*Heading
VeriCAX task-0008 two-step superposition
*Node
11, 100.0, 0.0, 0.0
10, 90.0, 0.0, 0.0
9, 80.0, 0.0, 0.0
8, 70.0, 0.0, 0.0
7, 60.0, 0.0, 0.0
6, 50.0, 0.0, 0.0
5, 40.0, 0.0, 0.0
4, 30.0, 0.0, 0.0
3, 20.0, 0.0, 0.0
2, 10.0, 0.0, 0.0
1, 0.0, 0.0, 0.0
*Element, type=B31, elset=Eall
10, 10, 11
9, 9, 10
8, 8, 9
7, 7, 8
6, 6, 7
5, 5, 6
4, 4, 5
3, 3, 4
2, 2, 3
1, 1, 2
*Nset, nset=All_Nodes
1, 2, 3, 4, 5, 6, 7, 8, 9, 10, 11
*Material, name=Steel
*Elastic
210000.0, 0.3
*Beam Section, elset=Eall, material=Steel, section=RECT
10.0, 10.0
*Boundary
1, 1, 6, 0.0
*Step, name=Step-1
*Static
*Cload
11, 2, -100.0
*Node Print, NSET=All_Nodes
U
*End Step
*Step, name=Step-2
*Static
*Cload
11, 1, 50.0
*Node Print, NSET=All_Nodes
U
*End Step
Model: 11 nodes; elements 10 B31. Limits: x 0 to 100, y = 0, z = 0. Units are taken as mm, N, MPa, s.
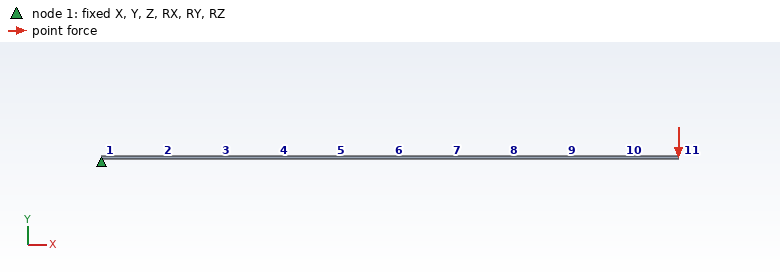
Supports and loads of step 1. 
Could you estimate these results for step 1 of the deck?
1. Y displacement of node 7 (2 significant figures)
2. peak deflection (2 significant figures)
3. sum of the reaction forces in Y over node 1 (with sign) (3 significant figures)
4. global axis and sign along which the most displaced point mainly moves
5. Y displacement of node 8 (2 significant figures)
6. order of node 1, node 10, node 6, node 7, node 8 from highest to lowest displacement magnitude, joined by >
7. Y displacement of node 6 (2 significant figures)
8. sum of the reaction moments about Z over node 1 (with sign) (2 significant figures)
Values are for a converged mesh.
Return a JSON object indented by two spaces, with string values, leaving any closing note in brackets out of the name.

{
  "Y displacement of node 7": "-0.083 mm",
  "peak deflection": "0.19 mm",
  "sum of the reaction forces in Y over node 1 (with sign)": "100 N",
  "global axis and sign along which the most displaced point mainly moves": "-Y",
  "Y displacement of node 8": "-0.11 mm",
  "order of node 1, node 10, node 6, node 7, node 8 from highest to lowest displacement magnitude, joined by >": "node 10 > node 8 > node 7 > node 6 > node 1",
  "Y displacement of node 6": "-0.060 mm",
  "sum of the reaction moments about Z over node 1 (with sign)": "10000 N·mm"
}
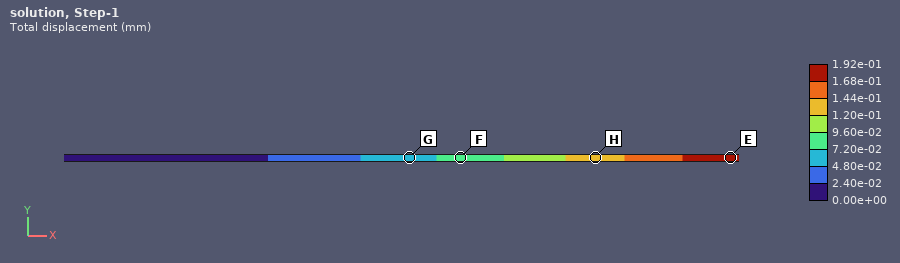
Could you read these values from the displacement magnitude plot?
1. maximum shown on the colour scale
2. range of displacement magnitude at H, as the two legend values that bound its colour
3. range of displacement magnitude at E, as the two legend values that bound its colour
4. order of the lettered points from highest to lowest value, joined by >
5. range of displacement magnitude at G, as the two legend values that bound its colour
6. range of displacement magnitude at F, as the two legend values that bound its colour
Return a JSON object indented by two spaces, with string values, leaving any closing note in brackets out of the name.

{
  "maximum shown on the colour scale": "1.92e-01 mm",
  "range of displacement magnitude at H, as the two legend values that bound its colour": "1.20e-01 to 1.44e-01 mm",
  "range of displacement magnitude at E, as the two legend values that bound its colour": "1.68e-01 to 1.92e-01 mm",
  "order of the lettered points from highest to lowest value, joined by >": "E > H > F > G",
  "range of displacement magnitude at G, as the two legend values that bound its colour": "4.80e-02 to 7.20e-02 mm",
  "range of displacement magnitude at F, as the two legend values that bound its colour": "7.20e-02 to 9.60e-02 mm"
}
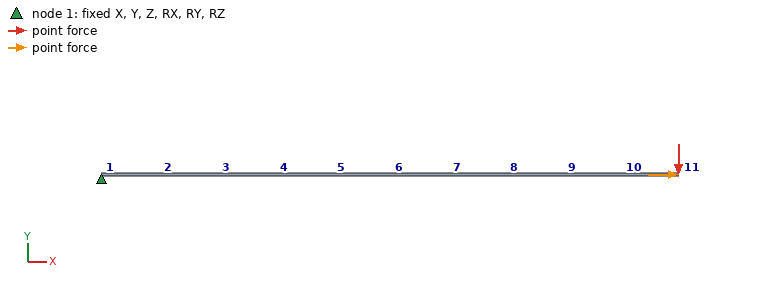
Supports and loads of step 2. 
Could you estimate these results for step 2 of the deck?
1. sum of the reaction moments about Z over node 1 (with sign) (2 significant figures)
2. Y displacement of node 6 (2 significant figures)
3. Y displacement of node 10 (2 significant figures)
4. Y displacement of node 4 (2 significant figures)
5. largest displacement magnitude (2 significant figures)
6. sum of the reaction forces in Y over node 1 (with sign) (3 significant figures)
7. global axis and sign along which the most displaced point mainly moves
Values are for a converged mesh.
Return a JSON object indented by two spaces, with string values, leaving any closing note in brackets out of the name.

{
  "sum of the reaction moments about Z over node 1 (with sign)": "10000 N·mm",
  "Y displacement of node 6": "-0.060 mm",
  "Y displacement of node 10": "-0.16 mm",
  "Y displacement of node 4": "-0.024 mm",
  "largest displacement magnitude": "0.19 mm",
  "sum of the reaction forces in Y over node 1 (with sign)": "100 N",
  "global axis and sign along which the most displaced point mainly moves": "-Y"
}
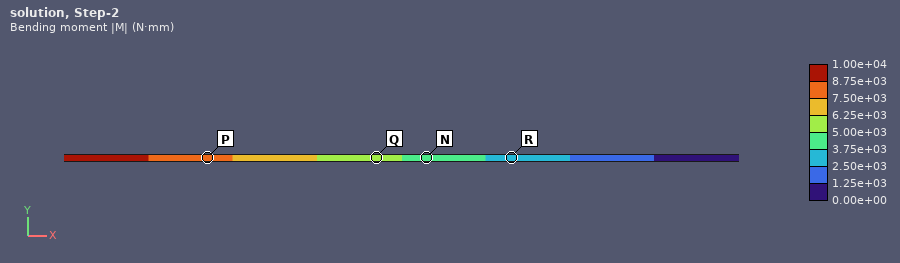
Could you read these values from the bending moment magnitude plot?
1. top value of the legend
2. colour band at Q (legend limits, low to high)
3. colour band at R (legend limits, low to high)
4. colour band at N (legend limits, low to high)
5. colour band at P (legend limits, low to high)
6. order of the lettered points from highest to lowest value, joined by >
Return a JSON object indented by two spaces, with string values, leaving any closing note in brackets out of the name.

{
  "top value of the legend": "1.00e+04 N·mm",
  "colour band at Q": "5.00e+03 to 6.25e+03 N·mm",
  "colour band at R": "2.50e+03 to 3.75e+03 N·mm",
  "colour band at N": "3.75e+03 to 5.00e+03 N·mm",
  "colour band at P": "7.50e+03 to 8.75e+03 N·mm",
  "order of the lettered points from highest to lowest value, joined by >": "P > Q > N > R"
}
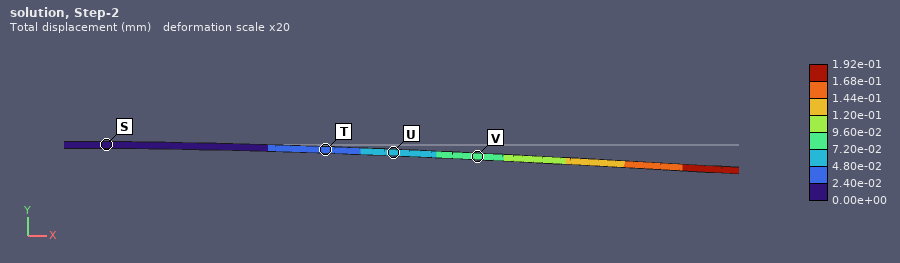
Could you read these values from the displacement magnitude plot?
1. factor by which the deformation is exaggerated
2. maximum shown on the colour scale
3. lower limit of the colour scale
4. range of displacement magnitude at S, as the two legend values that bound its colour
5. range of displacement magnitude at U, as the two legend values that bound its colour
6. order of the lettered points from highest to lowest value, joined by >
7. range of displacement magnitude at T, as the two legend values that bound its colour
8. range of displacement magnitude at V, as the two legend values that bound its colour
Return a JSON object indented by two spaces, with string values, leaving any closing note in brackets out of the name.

{
  "factor by which the deformation is exaggerated": "20",
  "maximum shown on the colour scale": "1.92e-01 mm",
  "lower limit of the colour scale": "0.00e+00 mm",
  "range of displacement magnitude at S, as the two legend values that bound its colour": "0.00e+00 to 2.40e-02 mm",
  "range of displacement magnitude at U, as the two legend values that bound its colour": "4.80e-02 to 7.20e-02 mm",
  "order of the lettered points from highest to lowest value, joined by >": "V > U > T > S",
  "range of displacement magnitude at T, as the two legend values that bound its colour": "2.40e-02 to 4.80e-02 mm",
  "range of displacement magnitude at V, as the two legend values that bound its colour": "7.20e-02 to 9.60e-02 mm"
}
